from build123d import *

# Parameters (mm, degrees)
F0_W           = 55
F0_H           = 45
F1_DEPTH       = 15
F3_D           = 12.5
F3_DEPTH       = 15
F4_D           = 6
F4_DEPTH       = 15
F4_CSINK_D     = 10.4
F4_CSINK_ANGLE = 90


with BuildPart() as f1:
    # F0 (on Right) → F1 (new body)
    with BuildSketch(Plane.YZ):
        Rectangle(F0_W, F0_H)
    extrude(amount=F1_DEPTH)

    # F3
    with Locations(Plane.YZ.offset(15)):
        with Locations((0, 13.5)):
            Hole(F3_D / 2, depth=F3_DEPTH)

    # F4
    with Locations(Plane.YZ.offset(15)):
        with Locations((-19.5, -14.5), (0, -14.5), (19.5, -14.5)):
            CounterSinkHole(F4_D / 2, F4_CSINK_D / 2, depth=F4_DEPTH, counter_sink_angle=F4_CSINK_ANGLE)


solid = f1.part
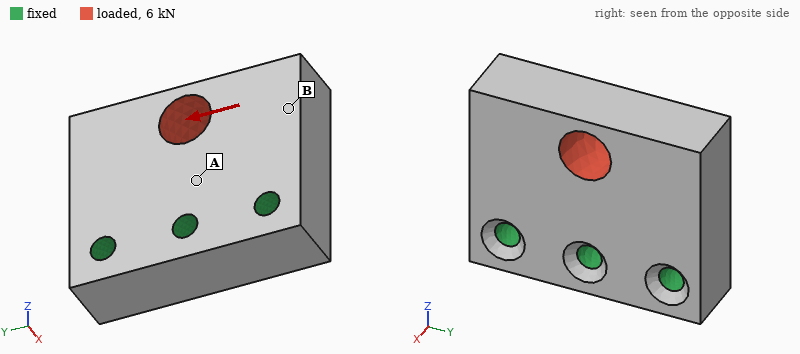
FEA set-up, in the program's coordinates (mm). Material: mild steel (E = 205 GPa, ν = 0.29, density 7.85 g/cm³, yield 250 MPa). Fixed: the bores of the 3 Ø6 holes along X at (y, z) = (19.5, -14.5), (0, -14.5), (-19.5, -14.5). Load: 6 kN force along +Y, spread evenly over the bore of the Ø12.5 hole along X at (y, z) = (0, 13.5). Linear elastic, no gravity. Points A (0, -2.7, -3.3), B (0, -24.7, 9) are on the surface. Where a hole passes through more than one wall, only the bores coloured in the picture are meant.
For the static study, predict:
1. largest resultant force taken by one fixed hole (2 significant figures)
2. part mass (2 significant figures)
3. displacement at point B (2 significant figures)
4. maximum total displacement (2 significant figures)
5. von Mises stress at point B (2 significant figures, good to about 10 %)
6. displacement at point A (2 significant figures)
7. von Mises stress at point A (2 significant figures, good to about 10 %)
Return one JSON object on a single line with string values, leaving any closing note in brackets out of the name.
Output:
{"largest resultant force taken by one fixed hole": "4.2 kN", "part mass": "270 g", "displacement at point B": "3.9 µm", "maximum total displacement": "6.3 µm", "von Mises stress at point B": "7.1 MPa", "displacement at point A": "1.4 µm", "von Mises stress at point A": "21 MPa"}
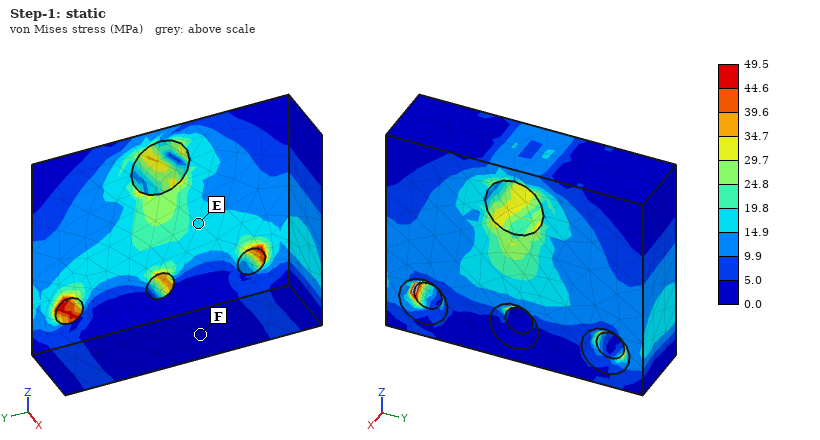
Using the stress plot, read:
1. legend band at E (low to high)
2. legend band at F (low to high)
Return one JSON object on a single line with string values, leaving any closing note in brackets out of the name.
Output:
{"legend band at E": "14.9 to 19.8 MPa", "legend band at F": "0.0 to 5.0 MPa"}
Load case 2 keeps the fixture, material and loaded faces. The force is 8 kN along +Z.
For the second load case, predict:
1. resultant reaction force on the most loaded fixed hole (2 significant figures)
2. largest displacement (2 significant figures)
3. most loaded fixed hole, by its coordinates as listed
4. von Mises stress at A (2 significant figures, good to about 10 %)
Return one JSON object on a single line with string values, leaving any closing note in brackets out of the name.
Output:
{"resultant reaction force on the most loaded fixed hole": "3.2 kN", "largest displacement": "5.5 µm", "most loaded fixed hole, by its coordinates as listed": "(0, -14.5)", "von Mises stress at A": "15 MPa"}
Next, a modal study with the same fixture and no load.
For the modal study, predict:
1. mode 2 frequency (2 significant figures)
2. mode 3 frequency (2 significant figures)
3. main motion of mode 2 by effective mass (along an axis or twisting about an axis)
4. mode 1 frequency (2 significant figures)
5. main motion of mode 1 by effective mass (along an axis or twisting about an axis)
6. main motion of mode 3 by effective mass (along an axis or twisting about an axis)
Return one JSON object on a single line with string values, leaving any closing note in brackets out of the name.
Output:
{"mode 2 frequency": "12 kHz", "mode 3 frequency": "16 kHz", "main motion of mode 2 by effective mass": "twisting about Z", "mode 1 frequency": "8100 Hz", "main motion of mode 1 by effective mass": "along X", "main motion of mode 3 by effective mass": "along Y"}
